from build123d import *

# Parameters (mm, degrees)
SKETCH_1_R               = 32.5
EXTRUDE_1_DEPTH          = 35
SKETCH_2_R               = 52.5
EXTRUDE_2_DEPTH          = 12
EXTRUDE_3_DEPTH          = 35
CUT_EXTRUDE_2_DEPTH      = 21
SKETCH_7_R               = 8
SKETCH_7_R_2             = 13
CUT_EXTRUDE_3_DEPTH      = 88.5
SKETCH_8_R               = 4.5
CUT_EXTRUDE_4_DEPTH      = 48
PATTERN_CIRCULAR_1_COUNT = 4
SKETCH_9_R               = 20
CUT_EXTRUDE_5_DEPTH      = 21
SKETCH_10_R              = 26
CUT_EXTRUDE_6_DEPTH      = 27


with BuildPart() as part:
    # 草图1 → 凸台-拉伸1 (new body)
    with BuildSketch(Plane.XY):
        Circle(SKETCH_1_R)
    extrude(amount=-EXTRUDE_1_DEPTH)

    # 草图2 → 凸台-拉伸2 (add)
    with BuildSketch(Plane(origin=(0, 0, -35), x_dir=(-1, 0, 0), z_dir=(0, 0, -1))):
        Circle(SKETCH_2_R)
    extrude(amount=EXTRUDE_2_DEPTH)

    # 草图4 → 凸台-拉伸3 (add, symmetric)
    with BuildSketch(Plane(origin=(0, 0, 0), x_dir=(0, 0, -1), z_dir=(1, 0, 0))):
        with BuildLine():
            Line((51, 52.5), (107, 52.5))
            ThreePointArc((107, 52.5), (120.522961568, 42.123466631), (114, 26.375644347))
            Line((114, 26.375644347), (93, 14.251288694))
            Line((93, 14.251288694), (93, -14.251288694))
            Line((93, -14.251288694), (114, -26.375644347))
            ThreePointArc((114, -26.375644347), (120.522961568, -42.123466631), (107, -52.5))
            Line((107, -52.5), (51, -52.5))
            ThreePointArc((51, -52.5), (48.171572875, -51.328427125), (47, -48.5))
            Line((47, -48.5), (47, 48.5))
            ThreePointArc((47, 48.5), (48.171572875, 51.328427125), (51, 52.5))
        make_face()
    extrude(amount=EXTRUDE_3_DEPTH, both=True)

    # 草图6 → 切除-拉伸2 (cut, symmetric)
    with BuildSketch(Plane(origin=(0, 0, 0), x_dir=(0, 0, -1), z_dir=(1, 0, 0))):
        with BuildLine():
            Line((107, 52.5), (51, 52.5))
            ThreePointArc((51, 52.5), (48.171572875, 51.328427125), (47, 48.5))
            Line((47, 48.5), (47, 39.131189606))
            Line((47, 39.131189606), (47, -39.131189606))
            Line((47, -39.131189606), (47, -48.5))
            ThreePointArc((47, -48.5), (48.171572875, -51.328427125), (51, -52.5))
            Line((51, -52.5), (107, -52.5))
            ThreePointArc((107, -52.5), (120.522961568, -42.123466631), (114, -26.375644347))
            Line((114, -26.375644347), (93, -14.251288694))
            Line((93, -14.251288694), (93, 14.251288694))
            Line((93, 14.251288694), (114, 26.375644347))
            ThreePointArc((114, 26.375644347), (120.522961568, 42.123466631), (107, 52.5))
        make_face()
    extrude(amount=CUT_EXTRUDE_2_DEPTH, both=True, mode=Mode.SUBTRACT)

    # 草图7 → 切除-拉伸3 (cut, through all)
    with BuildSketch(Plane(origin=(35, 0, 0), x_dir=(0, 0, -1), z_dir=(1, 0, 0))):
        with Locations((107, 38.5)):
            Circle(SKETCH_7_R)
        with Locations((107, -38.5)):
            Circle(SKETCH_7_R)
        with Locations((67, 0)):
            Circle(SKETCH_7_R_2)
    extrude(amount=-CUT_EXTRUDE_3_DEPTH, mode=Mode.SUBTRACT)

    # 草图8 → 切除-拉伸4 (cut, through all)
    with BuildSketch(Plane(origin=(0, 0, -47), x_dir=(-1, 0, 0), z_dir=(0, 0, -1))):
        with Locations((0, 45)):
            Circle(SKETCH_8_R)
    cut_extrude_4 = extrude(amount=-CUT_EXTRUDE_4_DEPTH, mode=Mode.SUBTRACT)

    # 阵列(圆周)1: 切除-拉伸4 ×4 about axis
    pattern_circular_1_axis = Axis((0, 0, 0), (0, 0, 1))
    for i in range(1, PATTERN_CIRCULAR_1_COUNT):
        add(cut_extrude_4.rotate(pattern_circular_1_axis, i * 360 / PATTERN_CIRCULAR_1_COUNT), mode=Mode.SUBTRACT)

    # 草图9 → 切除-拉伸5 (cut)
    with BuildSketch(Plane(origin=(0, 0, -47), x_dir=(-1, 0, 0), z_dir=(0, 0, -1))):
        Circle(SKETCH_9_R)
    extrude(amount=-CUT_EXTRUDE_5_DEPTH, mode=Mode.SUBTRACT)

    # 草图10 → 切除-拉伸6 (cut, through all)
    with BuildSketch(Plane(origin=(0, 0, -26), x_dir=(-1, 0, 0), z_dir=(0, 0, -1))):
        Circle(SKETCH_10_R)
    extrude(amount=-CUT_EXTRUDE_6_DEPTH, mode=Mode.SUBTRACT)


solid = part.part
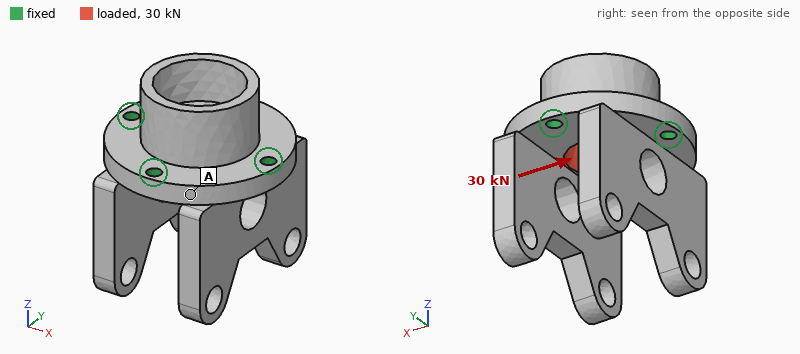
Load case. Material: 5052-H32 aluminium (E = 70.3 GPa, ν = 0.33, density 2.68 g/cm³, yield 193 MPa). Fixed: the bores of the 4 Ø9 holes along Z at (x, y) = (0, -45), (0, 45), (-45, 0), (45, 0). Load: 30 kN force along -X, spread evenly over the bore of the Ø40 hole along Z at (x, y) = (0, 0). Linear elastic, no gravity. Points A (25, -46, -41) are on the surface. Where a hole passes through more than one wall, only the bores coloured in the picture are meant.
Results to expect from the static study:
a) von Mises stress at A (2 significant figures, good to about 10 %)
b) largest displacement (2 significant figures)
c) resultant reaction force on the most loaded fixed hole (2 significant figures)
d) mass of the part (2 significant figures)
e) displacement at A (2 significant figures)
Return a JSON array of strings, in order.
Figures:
["9.4 MPa", "14 µm", "9.0 kN", "770 g", "5.5 µm"]
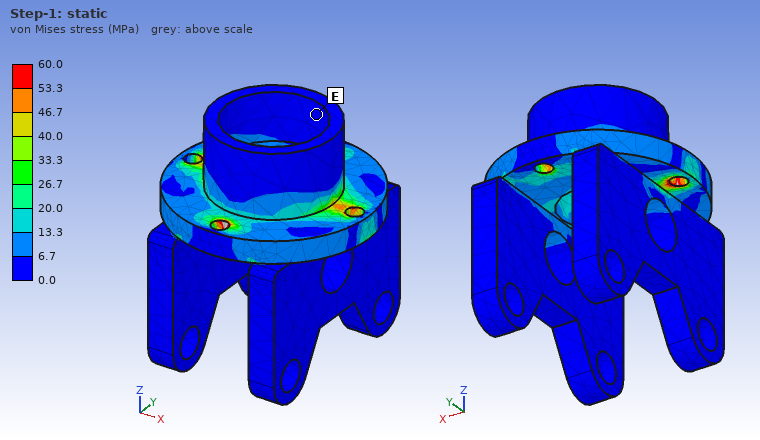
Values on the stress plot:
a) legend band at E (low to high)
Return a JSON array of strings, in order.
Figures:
["0.0 to 6.7 MPa"]
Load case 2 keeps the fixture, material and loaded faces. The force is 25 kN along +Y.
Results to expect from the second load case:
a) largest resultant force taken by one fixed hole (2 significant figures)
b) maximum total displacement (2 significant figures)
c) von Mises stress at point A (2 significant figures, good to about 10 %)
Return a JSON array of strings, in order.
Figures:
["7.4 kN", "12 µm", "8.5 MPa"]
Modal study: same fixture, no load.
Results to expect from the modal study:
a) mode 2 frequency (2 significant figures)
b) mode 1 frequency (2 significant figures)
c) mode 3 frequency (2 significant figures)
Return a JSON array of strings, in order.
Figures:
["2100 Hz", "2100 Hz", "2700 Hz"]
